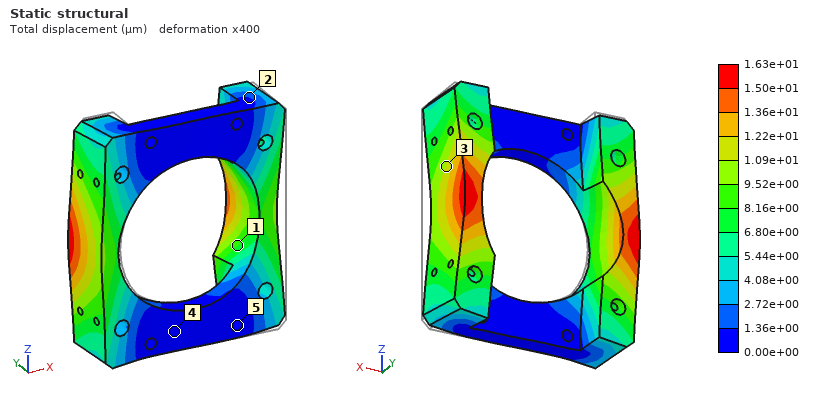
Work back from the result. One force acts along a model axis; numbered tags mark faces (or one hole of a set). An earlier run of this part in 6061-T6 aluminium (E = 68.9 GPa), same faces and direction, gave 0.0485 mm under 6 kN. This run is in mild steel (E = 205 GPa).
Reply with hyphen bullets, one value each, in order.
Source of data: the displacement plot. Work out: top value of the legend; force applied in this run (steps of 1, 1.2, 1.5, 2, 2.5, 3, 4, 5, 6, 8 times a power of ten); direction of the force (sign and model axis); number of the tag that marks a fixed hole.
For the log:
- 1.63e+01 µm
- 6 kN
- -X
- 5
